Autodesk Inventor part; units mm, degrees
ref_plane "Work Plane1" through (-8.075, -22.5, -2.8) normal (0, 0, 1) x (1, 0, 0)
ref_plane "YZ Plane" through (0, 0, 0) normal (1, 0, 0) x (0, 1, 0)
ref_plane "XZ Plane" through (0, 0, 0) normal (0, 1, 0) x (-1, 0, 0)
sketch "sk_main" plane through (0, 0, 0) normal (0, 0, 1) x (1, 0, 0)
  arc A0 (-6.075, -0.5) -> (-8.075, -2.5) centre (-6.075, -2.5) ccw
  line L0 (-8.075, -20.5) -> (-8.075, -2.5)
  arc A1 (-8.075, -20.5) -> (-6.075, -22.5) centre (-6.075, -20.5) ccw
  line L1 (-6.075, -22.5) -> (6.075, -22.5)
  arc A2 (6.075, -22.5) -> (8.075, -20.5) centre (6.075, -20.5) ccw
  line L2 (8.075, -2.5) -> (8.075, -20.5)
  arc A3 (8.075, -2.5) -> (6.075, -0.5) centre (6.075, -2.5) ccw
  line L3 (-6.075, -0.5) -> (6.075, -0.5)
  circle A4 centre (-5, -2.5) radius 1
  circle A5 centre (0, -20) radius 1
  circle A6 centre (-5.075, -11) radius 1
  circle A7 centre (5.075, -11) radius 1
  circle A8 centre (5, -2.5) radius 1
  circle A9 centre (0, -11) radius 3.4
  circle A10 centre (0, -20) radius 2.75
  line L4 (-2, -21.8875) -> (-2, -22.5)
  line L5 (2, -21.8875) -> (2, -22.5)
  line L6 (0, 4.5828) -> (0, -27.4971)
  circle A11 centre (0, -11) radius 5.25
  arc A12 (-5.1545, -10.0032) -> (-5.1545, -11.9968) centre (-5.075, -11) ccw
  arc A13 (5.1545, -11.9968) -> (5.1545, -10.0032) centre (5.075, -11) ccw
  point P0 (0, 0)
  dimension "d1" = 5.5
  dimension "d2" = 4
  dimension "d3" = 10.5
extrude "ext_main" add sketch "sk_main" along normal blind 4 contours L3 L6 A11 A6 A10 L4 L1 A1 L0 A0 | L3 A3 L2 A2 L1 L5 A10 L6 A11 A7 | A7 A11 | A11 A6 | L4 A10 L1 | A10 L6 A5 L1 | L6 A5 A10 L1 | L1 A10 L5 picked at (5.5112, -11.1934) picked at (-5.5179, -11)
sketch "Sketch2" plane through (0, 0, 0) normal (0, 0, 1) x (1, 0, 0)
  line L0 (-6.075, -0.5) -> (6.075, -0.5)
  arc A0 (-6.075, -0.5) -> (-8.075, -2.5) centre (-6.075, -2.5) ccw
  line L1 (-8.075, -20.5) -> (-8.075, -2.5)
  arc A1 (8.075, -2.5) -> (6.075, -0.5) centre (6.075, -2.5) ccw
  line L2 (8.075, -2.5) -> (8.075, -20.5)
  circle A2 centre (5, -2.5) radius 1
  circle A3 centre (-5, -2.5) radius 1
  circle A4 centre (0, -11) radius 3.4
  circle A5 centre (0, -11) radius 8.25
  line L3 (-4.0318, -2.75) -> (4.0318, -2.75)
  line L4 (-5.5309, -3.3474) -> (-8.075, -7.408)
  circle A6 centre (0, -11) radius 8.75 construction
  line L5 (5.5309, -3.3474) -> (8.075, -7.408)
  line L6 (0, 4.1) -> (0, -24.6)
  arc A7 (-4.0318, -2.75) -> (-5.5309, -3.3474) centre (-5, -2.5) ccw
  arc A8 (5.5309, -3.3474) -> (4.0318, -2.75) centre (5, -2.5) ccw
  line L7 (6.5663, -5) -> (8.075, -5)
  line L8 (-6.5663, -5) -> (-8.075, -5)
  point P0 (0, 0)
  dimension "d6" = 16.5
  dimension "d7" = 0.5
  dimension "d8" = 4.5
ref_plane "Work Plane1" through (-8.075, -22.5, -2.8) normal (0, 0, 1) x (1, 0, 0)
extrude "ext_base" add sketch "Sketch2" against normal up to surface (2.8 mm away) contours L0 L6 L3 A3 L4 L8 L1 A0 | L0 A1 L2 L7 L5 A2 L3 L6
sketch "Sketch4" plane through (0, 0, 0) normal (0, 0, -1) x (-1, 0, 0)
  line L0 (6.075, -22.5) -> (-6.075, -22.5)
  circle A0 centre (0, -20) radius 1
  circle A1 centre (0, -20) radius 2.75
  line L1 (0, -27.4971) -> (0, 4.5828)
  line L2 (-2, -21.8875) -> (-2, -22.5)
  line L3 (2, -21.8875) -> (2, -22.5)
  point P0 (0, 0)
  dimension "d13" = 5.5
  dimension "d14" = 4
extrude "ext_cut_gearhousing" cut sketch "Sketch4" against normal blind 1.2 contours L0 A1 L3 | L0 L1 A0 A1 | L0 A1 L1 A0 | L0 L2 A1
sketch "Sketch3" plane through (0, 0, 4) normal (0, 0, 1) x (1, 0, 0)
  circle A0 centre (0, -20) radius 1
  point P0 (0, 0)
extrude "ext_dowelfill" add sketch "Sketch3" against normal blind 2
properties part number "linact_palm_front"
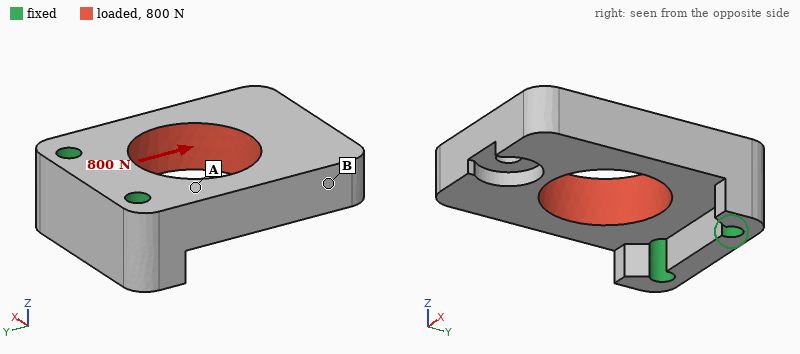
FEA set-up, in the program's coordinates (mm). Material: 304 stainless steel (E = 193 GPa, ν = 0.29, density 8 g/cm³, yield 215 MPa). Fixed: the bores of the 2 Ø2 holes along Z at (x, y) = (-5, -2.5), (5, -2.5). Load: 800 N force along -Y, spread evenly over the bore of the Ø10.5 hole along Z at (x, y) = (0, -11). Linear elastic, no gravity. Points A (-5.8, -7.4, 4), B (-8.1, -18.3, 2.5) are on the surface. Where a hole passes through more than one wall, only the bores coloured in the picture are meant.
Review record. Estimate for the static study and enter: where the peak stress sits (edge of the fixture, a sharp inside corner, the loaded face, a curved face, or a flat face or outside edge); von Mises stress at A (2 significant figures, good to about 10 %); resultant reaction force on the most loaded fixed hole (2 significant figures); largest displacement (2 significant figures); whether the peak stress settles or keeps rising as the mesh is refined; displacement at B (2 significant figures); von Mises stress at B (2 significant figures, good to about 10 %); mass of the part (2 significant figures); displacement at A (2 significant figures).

edge of the fixture
23 MPa
400 N
2.2 µm
keeps rising
1.2 µm
6.2 MPa
8.9 g
0.67 µm
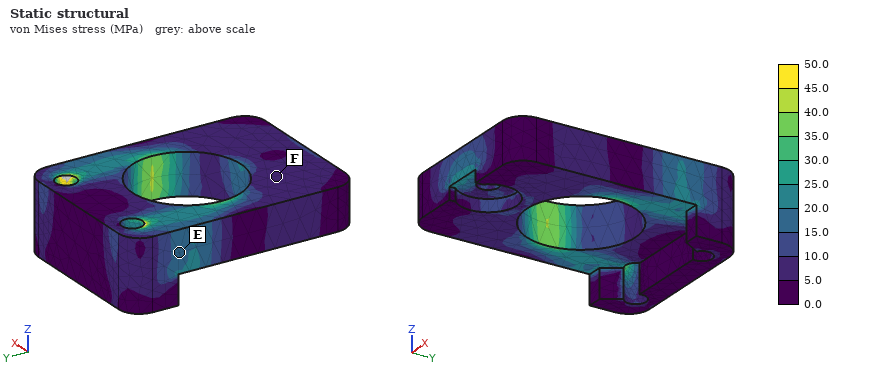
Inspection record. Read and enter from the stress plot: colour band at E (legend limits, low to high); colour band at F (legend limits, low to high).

15.0 to 20.0 MPa
5.0 to 10.0 MPa
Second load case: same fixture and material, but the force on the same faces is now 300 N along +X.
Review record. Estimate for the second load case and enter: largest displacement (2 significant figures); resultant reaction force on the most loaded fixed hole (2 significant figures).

5.5 µm
230 N
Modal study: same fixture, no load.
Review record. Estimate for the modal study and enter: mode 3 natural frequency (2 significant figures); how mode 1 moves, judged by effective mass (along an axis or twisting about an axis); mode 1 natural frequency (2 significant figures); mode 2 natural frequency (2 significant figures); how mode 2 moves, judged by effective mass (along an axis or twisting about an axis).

16 kHz
along Z
6400 Hz
14 kHz
along X
